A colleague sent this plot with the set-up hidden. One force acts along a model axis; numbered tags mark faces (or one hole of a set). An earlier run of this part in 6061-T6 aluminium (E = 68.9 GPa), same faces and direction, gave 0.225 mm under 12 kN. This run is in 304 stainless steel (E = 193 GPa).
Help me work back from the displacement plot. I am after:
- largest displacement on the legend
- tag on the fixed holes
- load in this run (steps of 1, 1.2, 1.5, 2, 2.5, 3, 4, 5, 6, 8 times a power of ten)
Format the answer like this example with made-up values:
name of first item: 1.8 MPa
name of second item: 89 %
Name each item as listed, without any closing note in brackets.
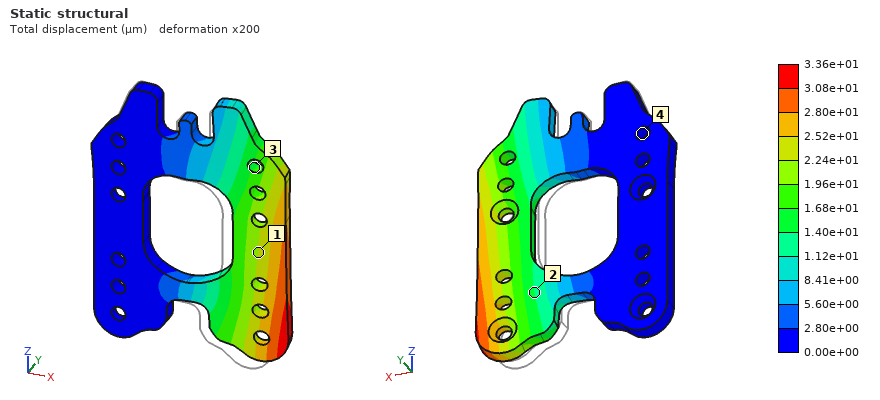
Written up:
largest displacement on the legend: 3.36e+01 µm
tag on the fixed holes: 4
load in this run: 5 kN
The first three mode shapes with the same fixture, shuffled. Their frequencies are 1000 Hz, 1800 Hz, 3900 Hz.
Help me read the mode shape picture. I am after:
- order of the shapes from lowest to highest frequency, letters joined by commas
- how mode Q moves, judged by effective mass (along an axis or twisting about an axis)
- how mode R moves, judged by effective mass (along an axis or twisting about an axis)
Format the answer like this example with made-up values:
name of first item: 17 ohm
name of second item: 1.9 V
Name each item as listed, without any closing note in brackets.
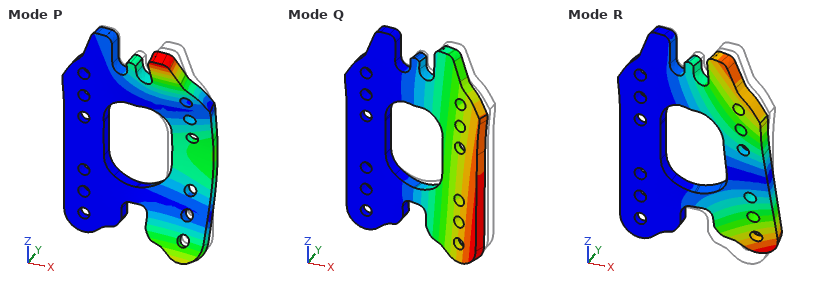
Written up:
order of the shapes from lowest to highest frequency, letters joined by commas: Q, R, P
how mode Q moves, judged by effective mass: along Y
how mode R moves, judged by effective mass: twisting about X
